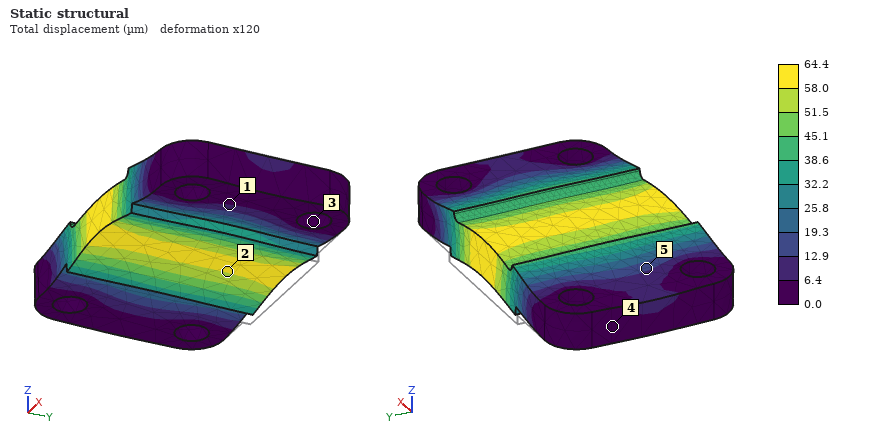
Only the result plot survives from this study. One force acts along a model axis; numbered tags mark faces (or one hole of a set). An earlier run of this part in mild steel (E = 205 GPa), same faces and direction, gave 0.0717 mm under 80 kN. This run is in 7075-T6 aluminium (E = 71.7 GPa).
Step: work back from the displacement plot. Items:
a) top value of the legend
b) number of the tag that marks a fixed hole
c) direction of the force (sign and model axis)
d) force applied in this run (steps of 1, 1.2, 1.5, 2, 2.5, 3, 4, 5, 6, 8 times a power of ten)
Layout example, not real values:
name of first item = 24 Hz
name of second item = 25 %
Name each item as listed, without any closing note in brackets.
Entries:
top value of the legend = 64.4 µm
number of the tag that marks a fixed hole = 3
direction of the force = +Z
force applied in this run = 25 kN
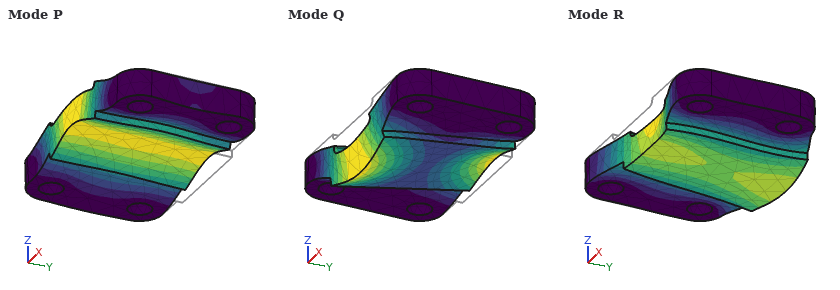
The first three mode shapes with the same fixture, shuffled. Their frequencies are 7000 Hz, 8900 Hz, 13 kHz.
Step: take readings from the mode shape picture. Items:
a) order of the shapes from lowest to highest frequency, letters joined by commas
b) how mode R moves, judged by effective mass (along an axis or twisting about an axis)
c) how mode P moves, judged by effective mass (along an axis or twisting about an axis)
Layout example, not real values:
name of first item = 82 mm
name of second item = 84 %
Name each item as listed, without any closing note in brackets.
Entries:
order of the shapes from lowest to highest frequency, letters joined by commas = P, Q, R
how mode R moves, judged by effective mass = along Y
how mode P moves, judged by effective mass = along Z
